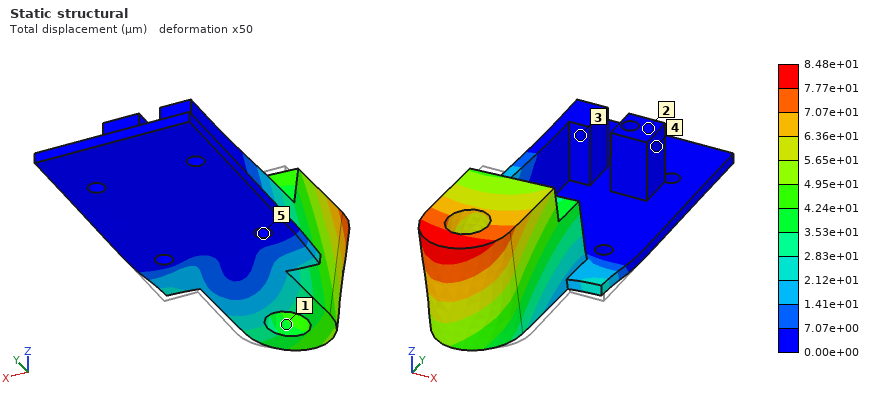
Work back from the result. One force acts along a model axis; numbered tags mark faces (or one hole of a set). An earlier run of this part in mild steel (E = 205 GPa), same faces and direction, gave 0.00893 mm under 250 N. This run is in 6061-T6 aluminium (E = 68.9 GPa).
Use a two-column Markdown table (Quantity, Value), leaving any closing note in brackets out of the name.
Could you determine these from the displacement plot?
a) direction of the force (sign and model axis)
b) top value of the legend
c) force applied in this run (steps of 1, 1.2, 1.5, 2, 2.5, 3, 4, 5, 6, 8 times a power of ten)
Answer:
| Quantity | Value |
|---|---|
| direction of the force | -X |
| top value of the legend | 8.48e+01 µm |
| force applied in this run | 800 N |
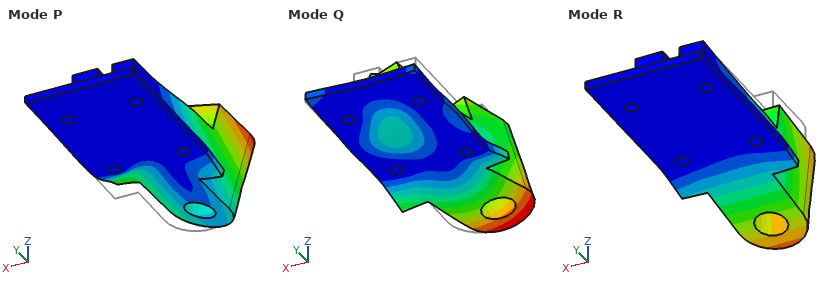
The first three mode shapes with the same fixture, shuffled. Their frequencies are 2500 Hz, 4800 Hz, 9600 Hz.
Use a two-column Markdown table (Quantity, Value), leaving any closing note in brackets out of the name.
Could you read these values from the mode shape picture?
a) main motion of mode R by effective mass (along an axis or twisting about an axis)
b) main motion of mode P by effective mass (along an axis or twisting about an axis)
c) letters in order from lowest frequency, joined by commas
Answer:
| Quantity | Value |
|---|---|
| main motion of mode R by effective mass | along Z |
| main motion of mode P by effective mass | along X |
| letters in order from lowest frequency, joined by commas | R, P, Q |
